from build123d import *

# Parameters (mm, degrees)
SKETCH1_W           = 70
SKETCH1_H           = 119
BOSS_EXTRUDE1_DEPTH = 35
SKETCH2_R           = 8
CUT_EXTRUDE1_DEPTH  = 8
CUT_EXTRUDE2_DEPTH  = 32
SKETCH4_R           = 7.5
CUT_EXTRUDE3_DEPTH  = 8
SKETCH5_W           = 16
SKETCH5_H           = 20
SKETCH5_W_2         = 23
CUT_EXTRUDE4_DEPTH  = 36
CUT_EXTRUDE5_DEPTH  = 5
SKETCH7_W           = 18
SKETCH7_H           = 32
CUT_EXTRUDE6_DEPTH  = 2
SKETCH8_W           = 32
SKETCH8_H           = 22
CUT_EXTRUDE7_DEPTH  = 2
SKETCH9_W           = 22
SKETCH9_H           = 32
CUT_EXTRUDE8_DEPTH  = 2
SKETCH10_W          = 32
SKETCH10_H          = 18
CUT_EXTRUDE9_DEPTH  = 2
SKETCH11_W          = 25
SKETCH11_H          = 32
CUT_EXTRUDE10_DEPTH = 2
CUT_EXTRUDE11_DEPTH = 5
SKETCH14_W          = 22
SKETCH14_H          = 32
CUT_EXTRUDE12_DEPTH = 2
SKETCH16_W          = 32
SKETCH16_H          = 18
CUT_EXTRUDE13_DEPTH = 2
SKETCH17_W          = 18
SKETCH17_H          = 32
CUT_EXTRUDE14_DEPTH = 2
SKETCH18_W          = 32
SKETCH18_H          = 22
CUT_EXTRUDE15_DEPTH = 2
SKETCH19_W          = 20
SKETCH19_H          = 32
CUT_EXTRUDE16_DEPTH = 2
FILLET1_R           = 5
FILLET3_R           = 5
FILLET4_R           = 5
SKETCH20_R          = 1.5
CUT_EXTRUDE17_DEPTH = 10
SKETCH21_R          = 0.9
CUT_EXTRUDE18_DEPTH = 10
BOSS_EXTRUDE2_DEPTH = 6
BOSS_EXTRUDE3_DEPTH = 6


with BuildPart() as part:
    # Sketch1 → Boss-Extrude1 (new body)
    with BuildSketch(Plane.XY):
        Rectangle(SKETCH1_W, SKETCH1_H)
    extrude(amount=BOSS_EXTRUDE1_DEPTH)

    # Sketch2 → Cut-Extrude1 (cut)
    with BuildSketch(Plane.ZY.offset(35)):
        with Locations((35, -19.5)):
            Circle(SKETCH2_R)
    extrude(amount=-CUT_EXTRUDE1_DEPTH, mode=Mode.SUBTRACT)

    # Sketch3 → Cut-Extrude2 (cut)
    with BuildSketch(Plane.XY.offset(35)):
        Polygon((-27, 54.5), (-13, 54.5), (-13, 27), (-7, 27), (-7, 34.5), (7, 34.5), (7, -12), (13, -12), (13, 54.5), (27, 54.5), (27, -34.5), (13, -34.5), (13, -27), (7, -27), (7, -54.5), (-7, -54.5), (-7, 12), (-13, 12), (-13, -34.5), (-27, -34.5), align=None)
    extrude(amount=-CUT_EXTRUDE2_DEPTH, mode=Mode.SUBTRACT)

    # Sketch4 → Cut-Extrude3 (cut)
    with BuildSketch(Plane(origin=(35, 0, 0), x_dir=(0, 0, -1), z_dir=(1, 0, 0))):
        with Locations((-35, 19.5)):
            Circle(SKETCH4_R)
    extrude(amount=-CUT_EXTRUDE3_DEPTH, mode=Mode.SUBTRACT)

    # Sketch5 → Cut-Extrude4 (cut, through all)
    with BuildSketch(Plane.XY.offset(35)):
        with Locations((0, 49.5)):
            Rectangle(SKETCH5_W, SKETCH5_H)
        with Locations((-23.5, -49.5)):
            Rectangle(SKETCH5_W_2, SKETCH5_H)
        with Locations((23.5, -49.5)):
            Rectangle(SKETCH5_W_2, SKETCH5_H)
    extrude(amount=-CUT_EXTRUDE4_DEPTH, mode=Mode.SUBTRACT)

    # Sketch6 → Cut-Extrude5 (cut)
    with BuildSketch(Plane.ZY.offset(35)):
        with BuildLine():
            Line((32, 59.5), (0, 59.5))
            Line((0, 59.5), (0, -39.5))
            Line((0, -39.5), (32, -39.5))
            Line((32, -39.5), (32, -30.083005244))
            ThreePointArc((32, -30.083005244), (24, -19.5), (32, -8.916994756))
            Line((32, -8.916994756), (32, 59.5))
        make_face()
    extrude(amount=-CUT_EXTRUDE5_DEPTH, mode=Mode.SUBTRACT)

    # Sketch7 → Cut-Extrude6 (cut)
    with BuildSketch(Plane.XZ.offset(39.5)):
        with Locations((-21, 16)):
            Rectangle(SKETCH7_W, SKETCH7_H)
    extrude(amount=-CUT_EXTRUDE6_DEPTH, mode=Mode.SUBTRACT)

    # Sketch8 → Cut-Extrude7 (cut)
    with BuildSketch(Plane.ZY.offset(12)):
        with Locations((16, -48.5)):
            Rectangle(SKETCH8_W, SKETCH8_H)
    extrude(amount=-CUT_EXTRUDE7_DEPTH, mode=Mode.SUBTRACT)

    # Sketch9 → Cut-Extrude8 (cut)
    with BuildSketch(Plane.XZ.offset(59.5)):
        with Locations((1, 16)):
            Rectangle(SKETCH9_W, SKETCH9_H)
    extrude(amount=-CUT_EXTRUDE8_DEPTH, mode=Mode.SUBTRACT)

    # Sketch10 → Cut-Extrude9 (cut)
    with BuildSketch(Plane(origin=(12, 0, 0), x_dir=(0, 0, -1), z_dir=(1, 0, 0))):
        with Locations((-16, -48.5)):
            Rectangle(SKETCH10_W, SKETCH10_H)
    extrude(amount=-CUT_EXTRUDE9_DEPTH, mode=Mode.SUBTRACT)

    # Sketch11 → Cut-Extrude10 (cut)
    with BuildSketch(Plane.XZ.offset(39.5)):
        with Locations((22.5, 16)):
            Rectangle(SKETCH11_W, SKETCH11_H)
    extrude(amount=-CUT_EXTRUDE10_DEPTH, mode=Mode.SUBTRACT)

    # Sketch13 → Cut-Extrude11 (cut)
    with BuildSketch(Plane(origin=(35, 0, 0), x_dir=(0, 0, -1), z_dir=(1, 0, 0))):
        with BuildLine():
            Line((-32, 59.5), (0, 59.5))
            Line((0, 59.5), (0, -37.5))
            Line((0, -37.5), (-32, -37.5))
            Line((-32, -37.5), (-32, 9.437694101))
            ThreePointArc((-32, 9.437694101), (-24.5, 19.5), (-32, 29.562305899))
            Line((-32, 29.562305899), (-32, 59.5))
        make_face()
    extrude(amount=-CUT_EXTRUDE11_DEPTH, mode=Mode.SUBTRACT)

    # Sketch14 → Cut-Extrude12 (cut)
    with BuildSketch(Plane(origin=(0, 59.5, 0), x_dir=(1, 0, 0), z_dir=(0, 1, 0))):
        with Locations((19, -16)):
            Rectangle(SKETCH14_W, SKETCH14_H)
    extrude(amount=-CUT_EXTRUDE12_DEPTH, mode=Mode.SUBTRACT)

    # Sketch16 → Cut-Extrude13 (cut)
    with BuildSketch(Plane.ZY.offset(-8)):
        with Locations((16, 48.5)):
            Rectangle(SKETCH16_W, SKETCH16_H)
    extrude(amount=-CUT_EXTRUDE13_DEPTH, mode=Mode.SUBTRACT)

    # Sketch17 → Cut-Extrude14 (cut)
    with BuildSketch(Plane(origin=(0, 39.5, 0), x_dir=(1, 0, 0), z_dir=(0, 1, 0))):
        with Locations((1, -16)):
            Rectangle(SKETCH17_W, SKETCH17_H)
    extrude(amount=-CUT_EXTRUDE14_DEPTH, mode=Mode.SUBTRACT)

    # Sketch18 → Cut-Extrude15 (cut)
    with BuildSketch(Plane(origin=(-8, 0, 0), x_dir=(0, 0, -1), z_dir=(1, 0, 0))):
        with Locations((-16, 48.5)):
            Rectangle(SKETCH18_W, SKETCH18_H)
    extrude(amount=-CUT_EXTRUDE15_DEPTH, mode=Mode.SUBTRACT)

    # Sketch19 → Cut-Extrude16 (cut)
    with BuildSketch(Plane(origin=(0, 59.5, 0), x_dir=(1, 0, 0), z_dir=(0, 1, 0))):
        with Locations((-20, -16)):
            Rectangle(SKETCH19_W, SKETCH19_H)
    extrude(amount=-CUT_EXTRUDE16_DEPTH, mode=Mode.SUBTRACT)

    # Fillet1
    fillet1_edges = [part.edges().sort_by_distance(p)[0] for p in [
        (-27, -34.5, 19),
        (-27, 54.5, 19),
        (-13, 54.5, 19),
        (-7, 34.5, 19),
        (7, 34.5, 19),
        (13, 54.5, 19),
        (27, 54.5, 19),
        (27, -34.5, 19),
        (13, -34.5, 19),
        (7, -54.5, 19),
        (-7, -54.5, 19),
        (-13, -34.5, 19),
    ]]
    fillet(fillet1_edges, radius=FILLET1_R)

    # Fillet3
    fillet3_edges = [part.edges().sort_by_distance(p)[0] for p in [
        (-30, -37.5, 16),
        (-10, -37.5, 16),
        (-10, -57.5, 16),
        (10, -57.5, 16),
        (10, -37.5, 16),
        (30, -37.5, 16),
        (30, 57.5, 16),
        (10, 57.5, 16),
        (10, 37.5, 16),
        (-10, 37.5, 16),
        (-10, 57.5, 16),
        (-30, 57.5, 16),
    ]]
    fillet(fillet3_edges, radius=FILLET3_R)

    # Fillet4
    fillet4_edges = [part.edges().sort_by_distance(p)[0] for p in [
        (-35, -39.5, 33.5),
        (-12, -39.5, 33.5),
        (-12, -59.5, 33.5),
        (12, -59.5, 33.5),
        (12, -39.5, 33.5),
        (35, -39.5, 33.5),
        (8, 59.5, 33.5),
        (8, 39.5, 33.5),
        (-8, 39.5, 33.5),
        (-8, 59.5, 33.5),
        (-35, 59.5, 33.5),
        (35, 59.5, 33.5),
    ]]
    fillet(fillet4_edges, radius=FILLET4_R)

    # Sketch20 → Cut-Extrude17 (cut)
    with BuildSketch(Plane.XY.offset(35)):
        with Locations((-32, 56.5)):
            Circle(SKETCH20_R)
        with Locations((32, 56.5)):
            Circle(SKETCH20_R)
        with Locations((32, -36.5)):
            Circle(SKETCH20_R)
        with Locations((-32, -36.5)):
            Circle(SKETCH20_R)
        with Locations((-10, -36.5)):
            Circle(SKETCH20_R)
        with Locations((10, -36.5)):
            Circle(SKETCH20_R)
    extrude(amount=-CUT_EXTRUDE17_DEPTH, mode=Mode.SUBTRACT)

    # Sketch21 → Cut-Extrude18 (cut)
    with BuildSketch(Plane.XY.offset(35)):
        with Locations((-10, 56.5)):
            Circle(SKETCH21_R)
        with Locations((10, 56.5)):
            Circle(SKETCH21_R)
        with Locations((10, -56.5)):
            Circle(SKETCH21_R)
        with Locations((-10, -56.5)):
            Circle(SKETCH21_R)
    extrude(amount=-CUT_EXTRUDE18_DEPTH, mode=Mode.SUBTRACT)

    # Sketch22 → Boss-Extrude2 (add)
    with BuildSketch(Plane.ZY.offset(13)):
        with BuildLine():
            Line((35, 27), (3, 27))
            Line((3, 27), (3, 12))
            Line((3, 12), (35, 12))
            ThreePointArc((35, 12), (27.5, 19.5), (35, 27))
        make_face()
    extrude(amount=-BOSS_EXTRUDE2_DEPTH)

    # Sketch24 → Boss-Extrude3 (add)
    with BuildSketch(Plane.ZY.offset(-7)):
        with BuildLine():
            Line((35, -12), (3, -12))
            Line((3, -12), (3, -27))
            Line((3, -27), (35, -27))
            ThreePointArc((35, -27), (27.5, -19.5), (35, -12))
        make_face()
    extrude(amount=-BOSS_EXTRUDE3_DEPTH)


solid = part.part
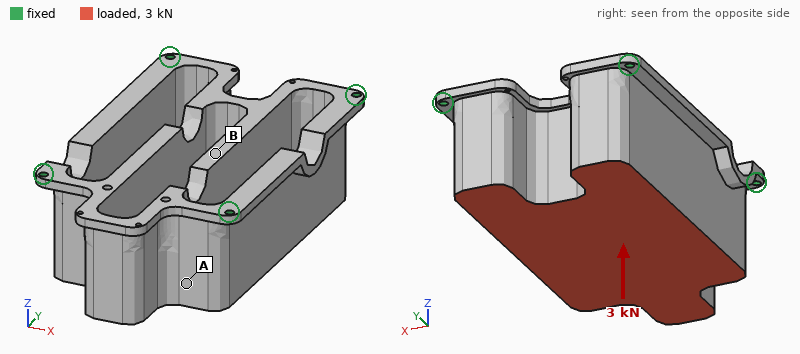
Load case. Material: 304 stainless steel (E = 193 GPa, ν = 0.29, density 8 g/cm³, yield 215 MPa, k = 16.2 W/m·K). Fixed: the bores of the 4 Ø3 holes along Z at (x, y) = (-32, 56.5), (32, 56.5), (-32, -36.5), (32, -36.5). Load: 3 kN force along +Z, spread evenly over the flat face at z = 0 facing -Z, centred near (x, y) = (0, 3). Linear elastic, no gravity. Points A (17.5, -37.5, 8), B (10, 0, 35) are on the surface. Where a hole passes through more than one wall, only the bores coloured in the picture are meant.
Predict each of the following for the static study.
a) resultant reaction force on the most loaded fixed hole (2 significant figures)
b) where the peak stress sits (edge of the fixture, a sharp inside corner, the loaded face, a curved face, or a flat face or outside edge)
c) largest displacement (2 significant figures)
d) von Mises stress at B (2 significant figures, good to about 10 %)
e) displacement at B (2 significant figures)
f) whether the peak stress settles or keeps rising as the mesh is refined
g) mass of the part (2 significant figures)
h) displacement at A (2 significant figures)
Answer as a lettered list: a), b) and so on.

a) 1.0 kN
b) edge of the fixture
c) 8.9 µm
d) 4.8 MPa
e) 8.2 µm
f) keeps rising
g) 670 g
h) 5.9 µm
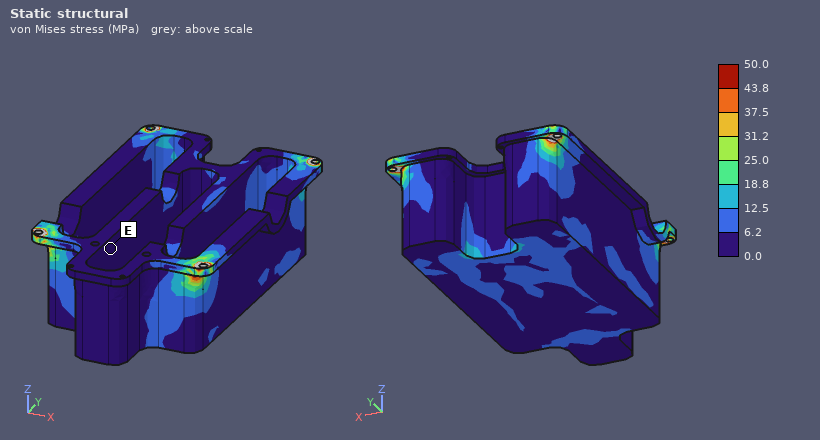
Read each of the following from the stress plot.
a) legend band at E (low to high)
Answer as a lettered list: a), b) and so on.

a) 0.0 to 6.2 MPa
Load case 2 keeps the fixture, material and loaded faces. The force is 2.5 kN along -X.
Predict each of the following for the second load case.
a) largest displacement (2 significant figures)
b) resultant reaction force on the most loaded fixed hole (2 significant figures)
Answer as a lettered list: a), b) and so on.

a) 15 µm
b) 1.2 kN
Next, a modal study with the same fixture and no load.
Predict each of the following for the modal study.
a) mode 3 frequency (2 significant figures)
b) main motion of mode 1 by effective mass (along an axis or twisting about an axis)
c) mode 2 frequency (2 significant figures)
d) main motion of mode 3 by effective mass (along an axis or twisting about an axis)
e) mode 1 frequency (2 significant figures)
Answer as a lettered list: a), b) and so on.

a) 4000 Hz
b) along X
c) 3600 Hz
d) along Z
e) 3100 Hz
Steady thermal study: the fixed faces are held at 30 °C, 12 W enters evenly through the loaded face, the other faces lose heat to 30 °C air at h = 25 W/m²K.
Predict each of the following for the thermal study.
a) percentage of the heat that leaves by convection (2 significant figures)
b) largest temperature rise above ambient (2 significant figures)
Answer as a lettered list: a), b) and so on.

a) 85 %
b) 17 K
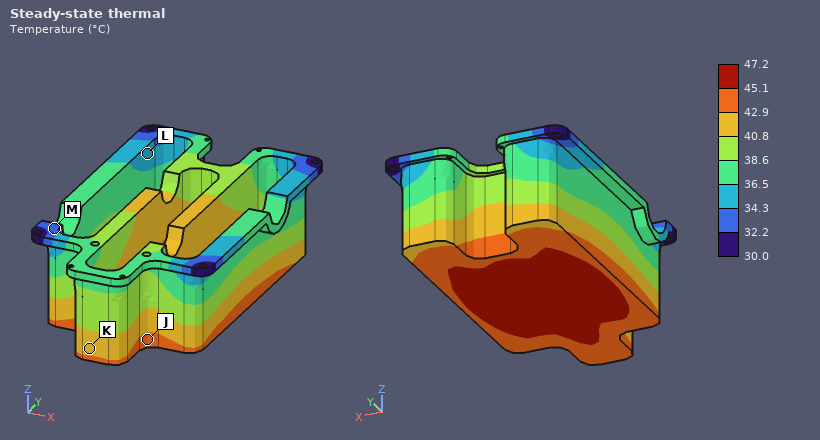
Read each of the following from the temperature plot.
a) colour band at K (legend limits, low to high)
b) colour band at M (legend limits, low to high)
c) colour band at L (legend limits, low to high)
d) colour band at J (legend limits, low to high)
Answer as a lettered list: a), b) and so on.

a) 40.8 to 42.9 °C
b) 32.2 to 34.3 °C
c) 34.3 to 36.5 °C
d) 42.9 to 45.1 °C
